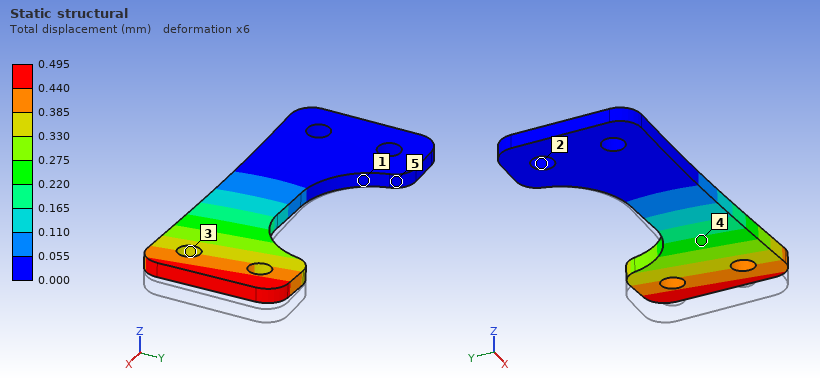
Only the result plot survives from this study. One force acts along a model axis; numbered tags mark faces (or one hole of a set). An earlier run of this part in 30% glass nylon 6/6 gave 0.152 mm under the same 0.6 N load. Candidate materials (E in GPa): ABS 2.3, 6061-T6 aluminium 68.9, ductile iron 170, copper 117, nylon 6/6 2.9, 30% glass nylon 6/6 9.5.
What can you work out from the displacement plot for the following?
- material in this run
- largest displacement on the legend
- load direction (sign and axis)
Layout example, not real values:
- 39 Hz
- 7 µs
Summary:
- nylon 6/6
- 0.495 mm
- +Z
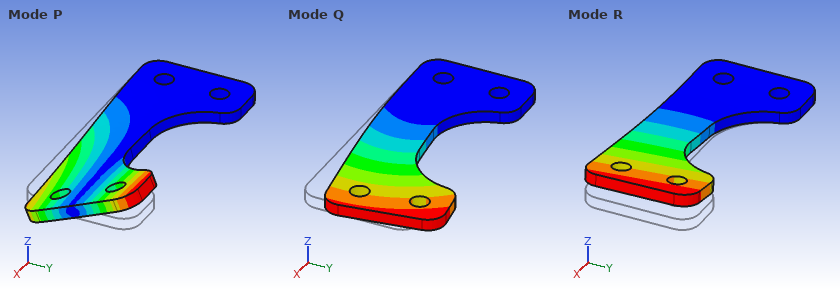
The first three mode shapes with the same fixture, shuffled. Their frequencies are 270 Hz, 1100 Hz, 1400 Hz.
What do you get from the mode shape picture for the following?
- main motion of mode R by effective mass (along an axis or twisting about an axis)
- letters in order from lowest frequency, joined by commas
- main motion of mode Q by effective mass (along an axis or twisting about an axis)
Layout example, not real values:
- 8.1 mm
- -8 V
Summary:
- along Z
- R, P, Q
- along Y
